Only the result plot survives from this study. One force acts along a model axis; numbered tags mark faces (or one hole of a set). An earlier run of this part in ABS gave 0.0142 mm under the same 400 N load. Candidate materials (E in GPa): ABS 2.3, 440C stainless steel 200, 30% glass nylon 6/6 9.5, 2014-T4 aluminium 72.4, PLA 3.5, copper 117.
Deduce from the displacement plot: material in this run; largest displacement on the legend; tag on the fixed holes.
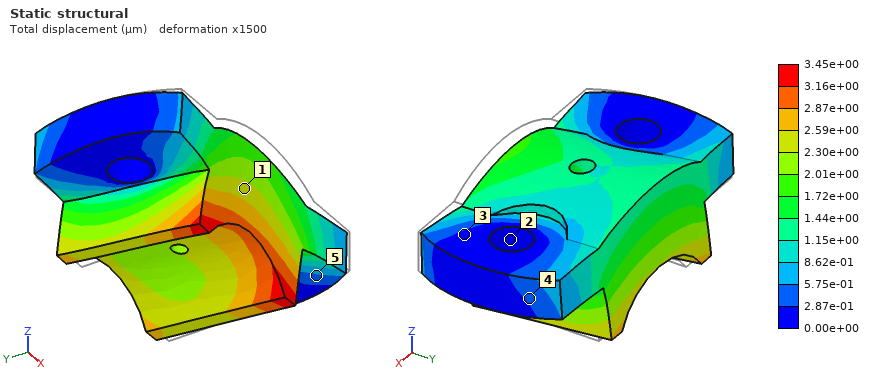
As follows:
30% glass nylon 6/6
3.45e+00 µm
2
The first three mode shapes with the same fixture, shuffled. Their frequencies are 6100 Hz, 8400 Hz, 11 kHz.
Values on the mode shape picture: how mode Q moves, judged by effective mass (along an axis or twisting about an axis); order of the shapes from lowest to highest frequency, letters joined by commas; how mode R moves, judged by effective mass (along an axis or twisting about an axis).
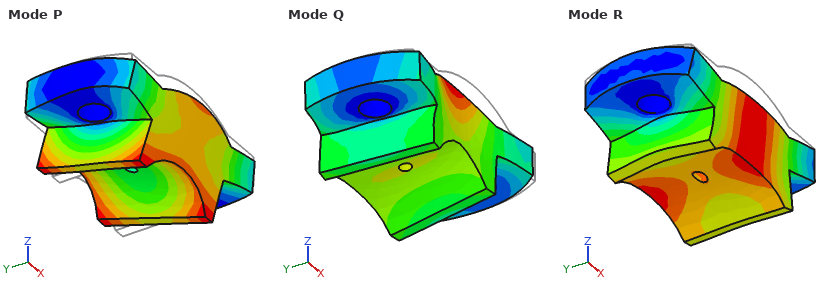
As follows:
along Y
P, R, Q
along Z
